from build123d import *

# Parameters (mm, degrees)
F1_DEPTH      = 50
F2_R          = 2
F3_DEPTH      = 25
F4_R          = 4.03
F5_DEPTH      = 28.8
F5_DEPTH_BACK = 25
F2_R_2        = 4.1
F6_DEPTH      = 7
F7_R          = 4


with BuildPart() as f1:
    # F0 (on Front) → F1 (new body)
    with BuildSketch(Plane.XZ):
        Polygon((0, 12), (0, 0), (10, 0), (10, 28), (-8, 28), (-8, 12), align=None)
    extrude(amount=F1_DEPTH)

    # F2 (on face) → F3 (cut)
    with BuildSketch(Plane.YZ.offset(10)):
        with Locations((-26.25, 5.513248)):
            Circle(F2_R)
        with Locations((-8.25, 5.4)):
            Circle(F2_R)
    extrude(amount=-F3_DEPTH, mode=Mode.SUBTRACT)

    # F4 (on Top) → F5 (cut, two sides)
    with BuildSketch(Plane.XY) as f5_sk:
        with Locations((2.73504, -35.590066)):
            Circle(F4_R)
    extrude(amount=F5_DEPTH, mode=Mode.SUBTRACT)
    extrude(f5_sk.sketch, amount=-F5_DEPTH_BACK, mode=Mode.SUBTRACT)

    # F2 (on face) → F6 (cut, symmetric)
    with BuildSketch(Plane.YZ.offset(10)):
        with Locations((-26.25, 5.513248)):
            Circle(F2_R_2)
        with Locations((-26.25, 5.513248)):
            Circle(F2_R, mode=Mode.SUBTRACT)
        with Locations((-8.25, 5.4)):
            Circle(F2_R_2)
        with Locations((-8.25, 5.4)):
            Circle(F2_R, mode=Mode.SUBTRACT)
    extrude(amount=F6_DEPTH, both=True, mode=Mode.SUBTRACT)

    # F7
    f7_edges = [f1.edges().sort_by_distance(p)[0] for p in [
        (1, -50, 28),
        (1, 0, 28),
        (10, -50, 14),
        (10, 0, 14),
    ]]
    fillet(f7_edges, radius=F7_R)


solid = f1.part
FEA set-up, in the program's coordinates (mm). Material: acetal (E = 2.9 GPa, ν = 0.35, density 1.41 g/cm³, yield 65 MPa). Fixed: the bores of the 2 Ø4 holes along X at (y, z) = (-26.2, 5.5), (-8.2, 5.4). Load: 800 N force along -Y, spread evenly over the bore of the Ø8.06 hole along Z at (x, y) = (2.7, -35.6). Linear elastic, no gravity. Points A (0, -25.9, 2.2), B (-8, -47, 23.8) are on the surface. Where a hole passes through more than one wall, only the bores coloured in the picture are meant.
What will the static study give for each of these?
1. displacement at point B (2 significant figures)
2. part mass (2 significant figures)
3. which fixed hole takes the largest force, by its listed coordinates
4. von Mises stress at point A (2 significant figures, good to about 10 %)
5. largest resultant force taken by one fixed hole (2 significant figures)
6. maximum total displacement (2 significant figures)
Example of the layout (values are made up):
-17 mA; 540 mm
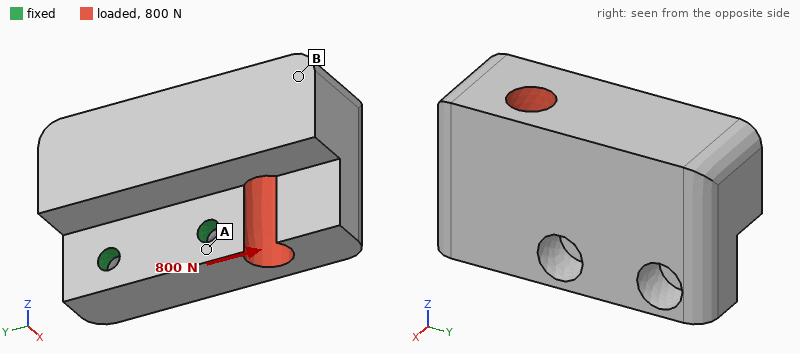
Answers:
0.12 mm; 25 g; (-26.2, 5.5); 4.8 MPa; 580 N; 0.13 mm
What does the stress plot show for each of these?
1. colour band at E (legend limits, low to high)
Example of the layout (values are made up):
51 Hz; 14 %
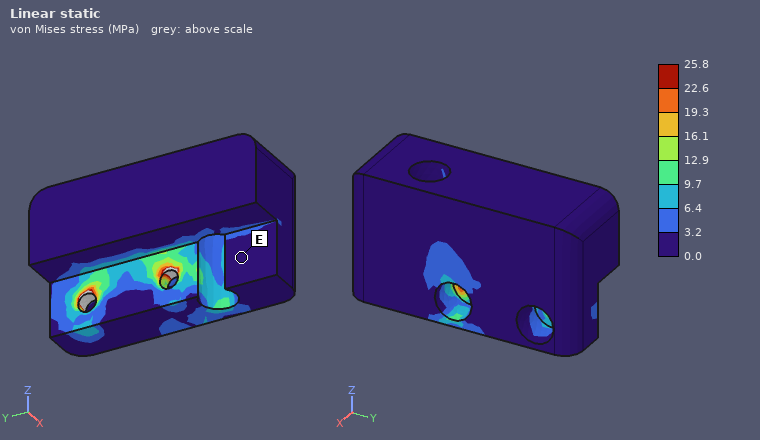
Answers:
0.0 to 3.2 MPa
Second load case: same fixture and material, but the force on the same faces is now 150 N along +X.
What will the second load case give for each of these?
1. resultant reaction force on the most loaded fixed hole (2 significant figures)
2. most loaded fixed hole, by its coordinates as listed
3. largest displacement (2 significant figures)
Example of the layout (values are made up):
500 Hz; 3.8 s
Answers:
210 N; (-26.2, 5.5); 0.29 mm
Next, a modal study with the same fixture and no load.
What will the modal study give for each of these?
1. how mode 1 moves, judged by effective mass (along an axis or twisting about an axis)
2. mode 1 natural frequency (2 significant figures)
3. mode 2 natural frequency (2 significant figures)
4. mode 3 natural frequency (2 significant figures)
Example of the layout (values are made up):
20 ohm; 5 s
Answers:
along X; 910 Hz; 1900 Hz; 2200 Hz
